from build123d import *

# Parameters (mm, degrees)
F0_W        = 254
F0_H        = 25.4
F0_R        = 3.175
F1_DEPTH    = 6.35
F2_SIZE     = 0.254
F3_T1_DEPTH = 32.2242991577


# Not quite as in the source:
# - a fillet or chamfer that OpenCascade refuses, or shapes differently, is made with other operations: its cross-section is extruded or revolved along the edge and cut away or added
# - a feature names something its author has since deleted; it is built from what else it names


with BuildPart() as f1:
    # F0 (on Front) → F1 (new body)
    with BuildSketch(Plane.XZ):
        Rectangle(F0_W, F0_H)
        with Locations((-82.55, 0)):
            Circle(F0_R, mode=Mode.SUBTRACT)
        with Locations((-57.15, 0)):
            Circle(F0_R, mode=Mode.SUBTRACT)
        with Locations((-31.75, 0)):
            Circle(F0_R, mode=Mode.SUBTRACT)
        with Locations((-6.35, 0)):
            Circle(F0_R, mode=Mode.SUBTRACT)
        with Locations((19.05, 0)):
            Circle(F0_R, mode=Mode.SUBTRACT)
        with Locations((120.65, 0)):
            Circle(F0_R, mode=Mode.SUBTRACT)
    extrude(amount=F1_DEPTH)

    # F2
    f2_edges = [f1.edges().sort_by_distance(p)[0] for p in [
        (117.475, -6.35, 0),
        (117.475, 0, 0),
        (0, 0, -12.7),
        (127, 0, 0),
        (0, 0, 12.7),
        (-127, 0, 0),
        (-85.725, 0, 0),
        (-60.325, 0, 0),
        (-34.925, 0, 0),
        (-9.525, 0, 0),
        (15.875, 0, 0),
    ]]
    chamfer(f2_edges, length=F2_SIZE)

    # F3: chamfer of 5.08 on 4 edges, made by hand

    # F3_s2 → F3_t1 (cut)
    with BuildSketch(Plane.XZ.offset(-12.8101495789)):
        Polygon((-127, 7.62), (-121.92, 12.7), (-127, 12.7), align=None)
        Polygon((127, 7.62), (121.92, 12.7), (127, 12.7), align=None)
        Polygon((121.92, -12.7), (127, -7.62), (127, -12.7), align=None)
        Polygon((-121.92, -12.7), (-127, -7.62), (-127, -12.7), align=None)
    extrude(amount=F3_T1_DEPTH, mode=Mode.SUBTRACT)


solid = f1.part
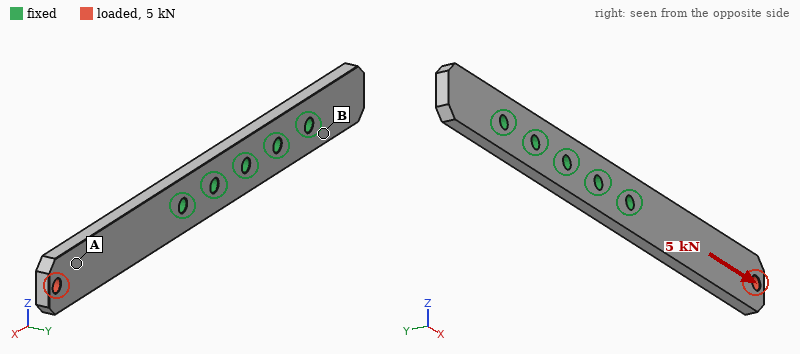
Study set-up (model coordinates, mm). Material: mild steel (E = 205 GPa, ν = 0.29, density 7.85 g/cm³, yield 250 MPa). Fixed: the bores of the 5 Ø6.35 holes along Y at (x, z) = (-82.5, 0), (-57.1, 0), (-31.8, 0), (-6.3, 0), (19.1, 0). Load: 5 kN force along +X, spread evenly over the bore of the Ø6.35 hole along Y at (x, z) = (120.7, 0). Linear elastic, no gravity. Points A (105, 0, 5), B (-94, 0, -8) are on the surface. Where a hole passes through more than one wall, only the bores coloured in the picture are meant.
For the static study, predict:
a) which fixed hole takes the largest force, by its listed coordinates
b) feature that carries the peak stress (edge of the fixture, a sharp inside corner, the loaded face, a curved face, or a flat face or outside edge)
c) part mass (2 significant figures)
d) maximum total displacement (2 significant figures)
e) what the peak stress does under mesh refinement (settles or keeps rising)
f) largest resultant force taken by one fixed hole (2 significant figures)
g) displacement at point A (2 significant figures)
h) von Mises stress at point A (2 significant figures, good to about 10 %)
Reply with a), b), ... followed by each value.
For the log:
a) (19.1, 0)
b) edge of the fixture
c) 310 g
d) 19 µm
e) keeps rising
f) 4.3 kN
g) 13 µm
h) 33 MPa
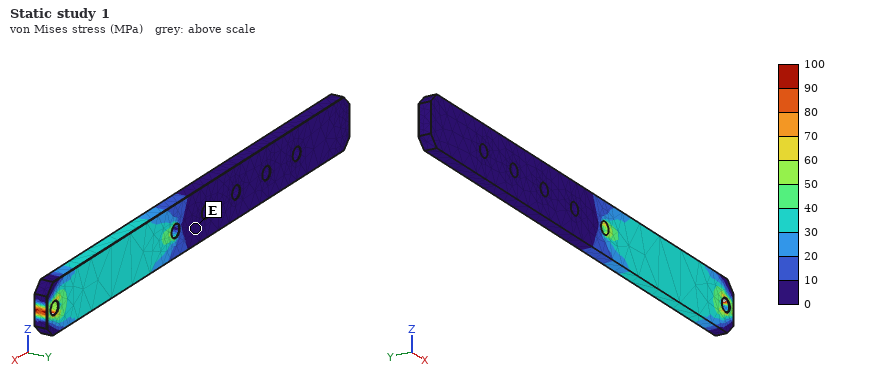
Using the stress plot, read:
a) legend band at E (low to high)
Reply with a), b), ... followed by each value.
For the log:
a) 0 to 10 MPa
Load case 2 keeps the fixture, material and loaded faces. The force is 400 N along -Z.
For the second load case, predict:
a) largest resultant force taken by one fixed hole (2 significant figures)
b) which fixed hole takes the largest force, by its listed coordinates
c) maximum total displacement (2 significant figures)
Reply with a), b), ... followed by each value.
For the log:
a) 1.3 kN
b) (19.1, 0)
c) 0.11 mm
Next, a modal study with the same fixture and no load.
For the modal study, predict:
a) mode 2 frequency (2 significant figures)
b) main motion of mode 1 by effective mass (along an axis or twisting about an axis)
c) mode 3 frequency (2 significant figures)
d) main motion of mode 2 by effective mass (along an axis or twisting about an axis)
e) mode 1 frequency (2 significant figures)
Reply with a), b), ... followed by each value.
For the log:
a) 1600 Hz
b) along Y
c) 2800 Hz
d) along Z
e) 470 Hz
